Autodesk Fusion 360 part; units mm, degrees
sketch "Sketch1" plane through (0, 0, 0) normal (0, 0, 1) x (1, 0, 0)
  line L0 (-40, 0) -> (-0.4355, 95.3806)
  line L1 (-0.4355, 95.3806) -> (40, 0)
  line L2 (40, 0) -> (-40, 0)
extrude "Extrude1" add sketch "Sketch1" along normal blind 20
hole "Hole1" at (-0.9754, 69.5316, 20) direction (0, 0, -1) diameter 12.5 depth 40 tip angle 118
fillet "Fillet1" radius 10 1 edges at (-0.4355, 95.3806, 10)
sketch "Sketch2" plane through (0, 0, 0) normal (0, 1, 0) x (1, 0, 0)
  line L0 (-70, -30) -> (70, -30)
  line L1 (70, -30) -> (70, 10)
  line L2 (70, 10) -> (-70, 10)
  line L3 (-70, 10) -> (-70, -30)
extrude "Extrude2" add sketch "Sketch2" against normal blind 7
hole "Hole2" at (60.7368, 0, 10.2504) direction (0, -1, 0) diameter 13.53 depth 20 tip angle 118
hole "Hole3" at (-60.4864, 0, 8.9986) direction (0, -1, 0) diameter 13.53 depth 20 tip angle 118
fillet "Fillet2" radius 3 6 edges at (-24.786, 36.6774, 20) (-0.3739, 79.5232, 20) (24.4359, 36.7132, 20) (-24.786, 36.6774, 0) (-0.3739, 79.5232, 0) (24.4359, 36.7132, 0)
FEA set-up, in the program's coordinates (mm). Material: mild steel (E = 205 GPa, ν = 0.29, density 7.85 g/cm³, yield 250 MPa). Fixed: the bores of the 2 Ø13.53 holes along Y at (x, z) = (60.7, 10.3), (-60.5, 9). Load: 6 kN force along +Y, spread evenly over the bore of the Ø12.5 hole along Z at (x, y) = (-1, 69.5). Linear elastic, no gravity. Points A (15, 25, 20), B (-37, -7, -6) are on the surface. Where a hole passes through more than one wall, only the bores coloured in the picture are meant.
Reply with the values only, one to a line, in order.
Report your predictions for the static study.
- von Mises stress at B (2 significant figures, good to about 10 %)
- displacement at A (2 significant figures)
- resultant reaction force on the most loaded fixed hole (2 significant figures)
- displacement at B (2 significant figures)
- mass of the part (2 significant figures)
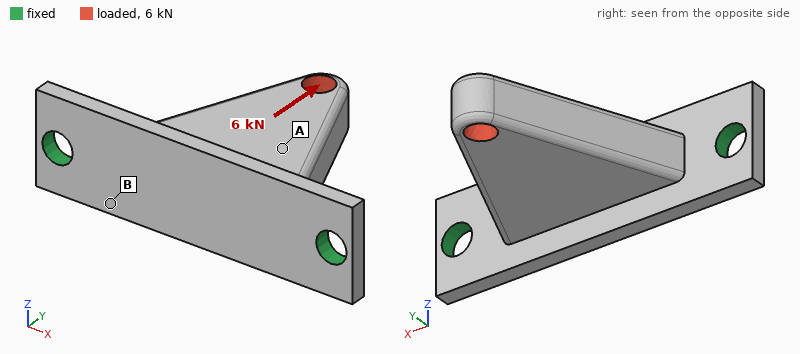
28 MPa
20 µm
3.6 kN
15 µm
850 g
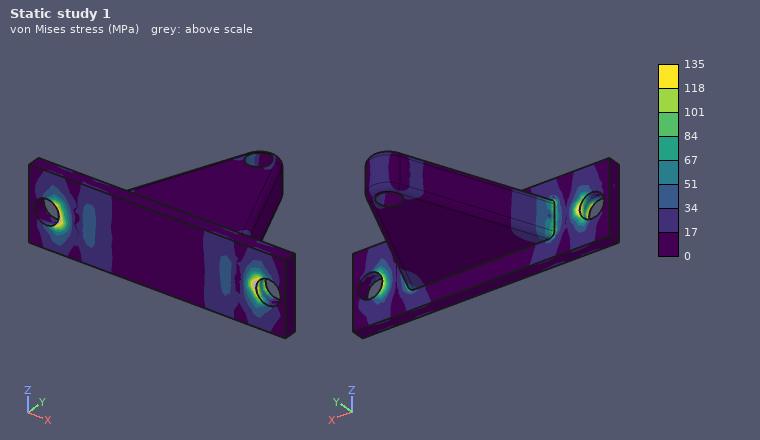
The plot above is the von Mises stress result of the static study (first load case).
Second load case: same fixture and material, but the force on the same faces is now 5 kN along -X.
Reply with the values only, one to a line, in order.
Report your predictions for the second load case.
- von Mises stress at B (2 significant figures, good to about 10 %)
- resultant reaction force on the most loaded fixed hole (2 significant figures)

48 MPa
4.6 kN
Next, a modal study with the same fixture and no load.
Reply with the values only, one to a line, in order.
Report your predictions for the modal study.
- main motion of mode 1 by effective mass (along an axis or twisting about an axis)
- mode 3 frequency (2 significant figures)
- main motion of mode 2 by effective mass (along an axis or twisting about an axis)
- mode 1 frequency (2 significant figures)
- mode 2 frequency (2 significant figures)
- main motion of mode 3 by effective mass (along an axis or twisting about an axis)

along Z
4000 Hz
along Y
1000 Hz
3300 Hz
along X
